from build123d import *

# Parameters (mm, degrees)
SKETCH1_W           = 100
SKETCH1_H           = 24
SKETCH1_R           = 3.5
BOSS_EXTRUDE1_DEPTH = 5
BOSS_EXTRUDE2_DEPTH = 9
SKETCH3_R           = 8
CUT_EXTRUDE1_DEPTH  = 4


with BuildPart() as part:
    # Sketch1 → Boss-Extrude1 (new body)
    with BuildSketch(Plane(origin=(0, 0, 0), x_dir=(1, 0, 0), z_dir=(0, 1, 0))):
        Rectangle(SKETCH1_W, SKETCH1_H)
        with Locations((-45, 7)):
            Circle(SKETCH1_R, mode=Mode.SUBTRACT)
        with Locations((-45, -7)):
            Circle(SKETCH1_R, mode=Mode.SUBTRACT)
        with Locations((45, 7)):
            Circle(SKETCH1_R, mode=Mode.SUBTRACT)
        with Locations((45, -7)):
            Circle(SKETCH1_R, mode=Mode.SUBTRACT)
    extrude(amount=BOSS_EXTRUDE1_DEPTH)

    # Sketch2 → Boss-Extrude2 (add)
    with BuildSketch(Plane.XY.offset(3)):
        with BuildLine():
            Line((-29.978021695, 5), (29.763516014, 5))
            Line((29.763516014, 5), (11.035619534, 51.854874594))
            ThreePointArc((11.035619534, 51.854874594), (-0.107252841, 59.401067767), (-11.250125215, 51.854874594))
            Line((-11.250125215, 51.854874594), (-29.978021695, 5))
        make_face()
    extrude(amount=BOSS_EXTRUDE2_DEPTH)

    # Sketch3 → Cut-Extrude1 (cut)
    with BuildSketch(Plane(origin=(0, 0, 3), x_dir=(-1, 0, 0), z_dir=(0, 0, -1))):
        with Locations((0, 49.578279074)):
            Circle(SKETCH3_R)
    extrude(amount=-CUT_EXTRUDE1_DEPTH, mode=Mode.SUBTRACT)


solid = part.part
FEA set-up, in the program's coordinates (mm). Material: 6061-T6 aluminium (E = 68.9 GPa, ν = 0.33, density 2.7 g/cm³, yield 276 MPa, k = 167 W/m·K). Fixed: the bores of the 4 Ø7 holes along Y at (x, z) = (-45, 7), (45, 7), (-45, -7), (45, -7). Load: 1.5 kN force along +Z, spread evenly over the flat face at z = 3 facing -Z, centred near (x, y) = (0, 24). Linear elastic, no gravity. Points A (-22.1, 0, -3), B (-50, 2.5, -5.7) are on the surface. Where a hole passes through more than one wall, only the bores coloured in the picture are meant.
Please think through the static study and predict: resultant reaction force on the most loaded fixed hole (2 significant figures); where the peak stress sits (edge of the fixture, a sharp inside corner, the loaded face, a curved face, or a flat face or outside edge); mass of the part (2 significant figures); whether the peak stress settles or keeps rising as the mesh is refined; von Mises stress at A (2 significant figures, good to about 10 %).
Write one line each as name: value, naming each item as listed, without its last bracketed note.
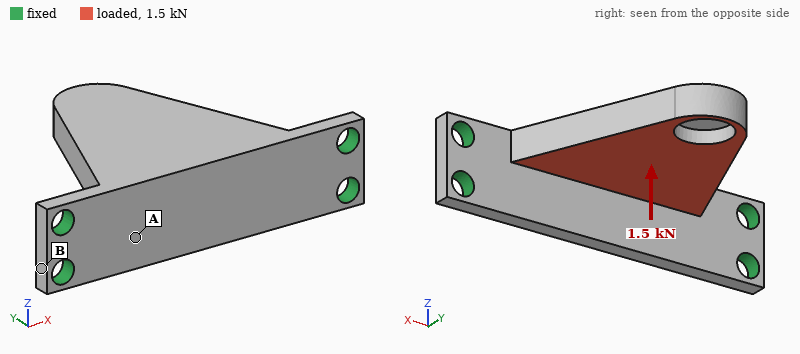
resultant reaction force on the most loaded fixed hole: 1.3 kN
where the peak stress sits: edge of the fixture
mass of the part: 78 g
whether the peak stress settles or keeps rising as the mesh is refined: keeps rising
von Mises stress at A: 64 MPa
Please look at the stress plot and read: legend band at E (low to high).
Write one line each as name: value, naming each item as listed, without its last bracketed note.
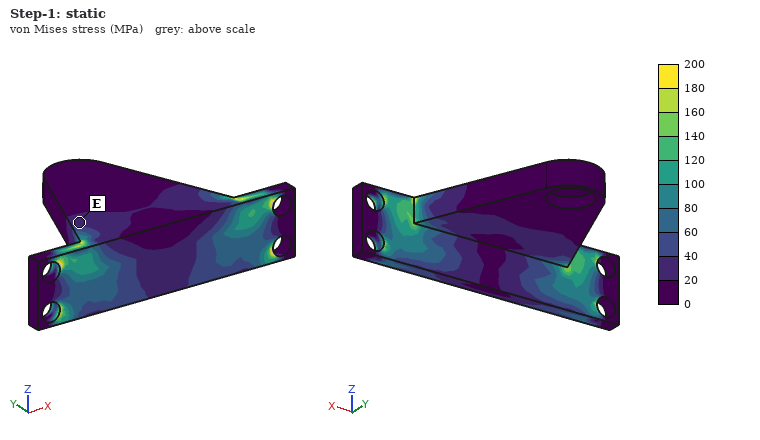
legend band at E: 20 to 40 MPa
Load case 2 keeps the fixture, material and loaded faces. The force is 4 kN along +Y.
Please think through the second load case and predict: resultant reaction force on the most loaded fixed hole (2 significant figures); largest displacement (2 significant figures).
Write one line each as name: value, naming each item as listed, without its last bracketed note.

resultant reaction force on the most loaded fixed hole: 1.8 kN
largest displacement: 0.18 mm
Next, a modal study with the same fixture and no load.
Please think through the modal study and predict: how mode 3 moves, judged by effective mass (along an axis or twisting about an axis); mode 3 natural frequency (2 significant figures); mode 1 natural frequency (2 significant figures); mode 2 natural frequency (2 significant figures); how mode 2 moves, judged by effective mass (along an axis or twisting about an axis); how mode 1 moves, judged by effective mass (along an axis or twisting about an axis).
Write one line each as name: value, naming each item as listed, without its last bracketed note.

how mode 3 moves, judged by effective mass: along X
mode 3 natural frequency: 5400 Hz
mode 1 natural frequency: 1400 Hz
mode 2 natural frequency: 4200 Hz
how mode 2 moves, judged by effective mass: along Y
how mode 1 moves, judged by effective mass: along Z
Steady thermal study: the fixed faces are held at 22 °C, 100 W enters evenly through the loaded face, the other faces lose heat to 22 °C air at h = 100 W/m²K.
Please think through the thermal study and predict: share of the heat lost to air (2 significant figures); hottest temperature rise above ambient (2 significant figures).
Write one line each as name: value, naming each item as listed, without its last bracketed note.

share of the heat lost to air: 31 %
hottest temperature rise above ambient: 62 K
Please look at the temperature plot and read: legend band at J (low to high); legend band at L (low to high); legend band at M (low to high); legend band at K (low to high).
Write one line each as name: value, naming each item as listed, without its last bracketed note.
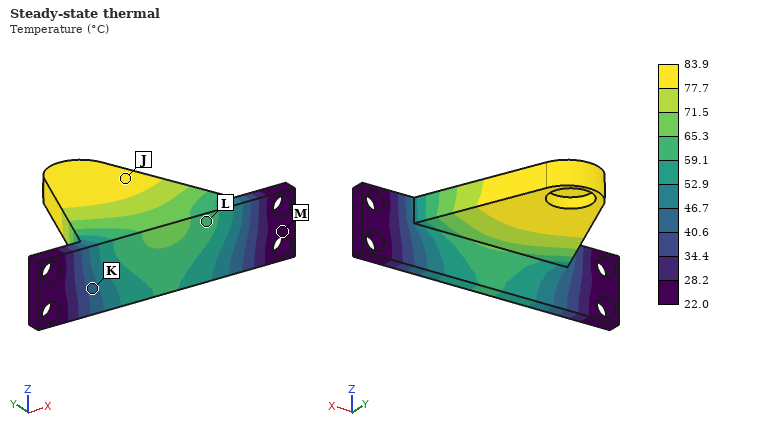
legend band at J: 77.7 to 83.9 °C
legend band at L: 59.1 to 65.3 °C
legend band at M: 22.0 to 28.2 °C
legend band at K: 40.6 to 46.7 °C
